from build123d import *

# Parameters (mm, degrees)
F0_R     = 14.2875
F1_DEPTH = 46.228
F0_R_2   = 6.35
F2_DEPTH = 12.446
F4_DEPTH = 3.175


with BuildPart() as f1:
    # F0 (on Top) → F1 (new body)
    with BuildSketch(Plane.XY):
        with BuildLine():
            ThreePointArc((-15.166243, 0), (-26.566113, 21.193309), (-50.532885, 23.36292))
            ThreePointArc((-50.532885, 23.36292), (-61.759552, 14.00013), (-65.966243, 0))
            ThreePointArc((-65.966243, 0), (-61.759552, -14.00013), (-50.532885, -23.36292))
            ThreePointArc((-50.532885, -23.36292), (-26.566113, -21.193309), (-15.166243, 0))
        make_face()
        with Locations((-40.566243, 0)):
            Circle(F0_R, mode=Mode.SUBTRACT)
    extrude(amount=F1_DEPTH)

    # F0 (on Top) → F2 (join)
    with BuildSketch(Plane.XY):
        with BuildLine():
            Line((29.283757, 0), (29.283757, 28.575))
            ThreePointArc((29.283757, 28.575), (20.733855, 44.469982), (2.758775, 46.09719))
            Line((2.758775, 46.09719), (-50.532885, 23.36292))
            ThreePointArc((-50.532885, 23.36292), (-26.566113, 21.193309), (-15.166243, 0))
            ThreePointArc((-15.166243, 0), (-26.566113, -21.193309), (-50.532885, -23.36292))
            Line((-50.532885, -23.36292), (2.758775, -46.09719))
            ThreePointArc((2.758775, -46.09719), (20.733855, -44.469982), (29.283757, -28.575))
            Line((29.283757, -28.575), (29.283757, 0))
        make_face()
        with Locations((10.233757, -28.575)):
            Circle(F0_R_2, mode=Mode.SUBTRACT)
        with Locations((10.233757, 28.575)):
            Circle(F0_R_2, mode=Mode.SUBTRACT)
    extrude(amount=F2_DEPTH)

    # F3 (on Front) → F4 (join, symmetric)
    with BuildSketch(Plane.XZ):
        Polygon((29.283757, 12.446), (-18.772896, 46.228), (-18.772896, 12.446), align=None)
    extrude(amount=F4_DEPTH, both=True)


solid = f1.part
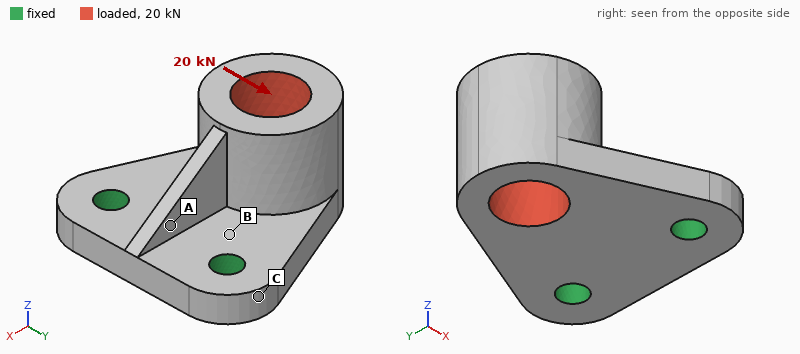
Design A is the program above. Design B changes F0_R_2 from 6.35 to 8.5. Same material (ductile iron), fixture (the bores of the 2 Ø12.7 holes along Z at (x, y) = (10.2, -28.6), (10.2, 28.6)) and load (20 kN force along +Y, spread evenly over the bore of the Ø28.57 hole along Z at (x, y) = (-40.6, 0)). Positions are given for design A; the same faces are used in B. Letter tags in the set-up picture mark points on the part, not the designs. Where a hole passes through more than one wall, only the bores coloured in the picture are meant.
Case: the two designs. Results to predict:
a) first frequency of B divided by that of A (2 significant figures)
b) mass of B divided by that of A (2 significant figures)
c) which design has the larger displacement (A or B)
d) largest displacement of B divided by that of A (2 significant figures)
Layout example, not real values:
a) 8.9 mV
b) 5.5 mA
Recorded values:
a) 1.1
b) 0.98
c) A
d) 0.91
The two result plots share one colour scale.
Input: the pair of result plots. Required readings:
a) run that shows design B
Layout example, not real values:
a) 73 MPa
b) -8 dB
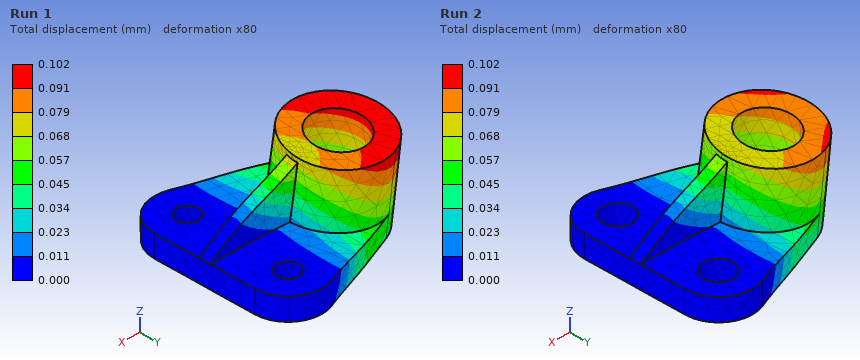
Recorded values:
a) Run 2
